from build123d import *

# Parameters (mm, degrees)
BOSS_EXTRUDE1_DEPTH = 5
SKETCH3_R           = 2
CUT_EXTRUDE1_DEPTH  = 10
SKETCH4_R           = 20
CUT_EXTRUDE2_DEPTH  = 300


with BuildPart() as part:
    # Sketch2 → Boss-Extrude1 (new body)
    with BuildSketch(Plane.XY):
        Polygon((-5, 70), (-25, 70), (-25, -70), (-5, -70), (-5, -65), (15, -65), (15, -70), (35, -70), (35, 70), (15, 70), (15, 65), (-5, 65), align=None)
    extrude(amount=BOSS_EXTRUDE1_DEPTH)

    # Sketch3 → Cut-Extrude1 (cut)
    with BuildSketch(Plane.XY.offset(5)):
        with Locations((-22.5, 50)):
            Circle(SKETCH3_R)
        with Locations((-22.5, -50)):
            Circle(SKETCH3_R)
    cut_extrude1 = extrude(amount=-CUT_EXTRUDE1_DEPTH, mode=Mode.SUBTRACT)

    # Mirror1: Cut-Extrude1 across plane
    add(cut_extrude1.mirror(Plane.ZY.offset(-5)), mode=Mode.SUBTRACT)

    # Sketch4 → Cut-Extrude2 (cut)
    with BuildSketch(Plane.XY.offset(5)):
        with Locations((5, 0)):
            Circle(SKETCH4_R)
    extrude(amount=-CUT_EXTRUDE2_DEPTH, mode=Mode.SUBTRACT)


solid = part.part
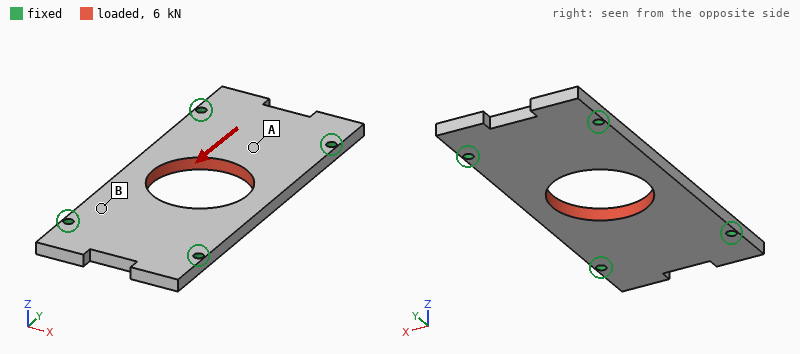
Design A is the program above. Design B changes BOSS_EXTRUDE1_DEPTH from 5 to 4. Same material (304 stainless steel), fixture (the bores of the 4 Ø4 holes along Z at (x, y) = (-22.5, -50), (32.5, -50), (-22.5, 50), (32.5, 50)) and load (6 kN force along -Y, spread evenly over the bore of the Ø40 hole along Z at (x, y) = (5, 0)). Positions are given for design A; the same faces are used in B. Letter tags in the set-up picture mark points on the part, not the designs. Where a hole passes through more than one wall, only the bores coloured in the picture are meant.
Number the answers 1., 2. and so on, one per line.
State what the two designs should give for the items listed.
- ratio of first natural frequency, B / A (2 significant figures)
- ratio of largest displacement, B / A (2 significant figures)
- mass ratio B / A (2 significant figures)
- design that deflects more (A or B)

1. 0.81
2. 1.3
3. 0.80
4. B
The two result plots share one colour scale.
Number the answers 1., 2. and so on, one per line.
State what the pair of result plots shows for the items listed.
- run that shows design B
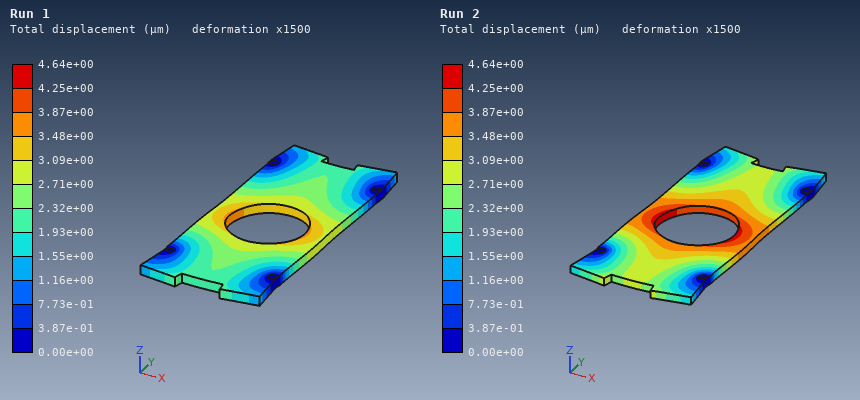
1. Run 2
